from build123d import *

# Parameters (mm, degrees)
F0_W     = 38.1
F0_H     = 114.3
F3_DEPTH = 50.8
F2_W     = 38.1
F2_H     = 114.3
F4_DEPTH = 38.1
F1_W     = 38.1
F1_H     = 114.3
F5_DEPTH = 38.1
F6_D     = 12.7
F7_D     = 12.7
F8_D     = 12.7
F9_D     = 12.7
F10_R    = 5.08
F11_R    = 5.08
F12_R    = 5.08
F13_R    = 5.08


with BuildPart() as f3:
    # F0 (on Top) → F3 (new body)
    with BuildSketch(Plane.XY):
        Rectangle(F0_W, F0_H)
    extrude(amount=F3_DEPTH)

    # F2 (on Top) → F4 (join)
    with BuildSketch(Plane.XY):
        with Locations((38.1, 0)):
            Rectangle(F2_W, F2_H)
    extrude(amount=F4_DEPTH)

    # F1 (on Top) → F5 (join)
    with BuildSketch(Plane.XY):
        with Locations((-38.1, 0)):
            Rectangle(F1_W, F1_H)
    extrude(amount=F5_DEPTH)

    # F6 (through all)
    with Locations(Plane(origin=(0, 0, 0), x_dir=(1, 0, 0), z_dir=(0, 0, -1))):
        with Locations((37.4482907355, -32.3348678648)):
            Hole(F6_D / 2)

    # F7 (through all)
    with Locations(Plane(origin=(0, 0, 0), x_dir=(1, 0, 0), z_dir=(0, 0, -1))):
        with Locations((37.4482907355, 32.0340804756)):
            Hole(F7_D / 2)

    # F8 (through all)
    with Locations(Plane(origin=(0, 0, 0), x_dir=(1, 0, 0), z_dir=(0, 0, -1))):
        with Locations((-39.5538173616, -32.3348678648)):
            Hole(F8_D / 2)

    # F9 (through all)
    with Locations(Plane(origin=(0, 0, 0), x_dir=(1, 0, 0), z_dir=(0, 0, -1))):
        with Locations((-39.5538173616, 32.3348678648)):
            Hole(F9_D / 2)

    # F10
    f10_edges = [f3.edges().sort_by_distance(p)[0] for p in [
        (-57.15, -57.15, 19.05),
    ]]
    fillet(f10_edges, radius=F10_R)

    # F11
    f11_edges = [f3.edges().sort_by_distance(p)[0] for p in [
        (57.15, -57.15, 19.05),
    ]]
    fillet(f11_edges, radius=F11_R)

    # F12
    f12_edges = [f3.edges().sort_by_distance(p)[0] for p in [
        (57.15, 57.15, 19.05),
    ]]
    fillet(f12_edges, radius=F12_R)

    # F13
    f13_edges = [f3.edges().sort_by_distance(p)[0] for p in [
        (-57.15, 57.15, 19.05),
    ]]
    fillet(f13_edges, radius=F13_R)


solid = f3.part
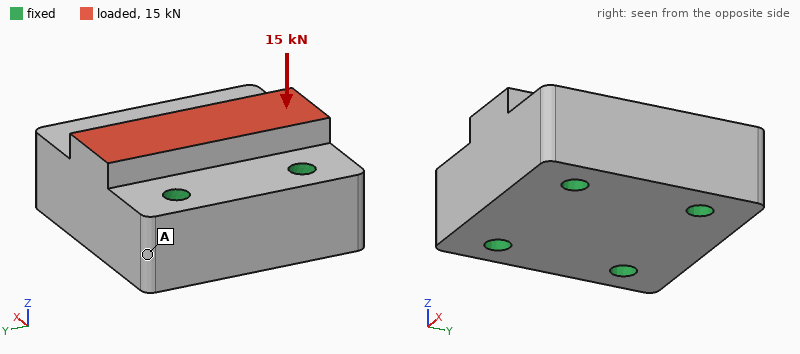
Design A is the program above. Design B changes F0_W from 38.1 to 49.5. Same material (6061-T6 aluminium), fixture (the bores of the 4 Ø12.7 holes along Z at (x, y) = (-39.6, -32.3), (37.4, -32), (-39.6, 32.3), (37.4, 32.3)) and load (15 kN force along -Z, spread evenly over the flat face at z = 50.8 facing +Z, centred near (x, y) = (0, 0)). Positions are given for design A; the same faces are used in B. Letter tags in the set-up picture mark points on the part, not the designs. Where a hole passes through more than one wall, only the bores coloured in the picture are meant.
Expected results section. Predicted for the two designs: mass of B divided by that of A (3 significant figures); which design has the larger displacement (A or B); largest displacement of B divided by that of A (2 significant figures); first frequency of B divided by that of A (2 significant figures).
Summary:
1.03
A
0.85
1.00
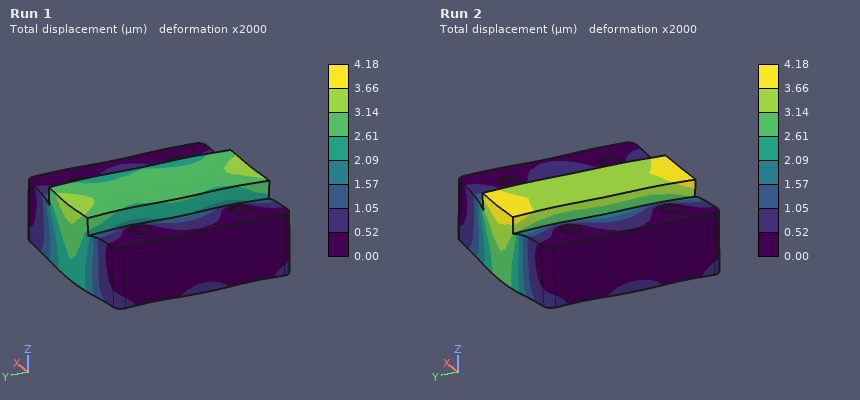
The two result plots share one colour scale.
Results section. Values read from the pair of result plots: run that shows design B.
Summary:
Run 1
